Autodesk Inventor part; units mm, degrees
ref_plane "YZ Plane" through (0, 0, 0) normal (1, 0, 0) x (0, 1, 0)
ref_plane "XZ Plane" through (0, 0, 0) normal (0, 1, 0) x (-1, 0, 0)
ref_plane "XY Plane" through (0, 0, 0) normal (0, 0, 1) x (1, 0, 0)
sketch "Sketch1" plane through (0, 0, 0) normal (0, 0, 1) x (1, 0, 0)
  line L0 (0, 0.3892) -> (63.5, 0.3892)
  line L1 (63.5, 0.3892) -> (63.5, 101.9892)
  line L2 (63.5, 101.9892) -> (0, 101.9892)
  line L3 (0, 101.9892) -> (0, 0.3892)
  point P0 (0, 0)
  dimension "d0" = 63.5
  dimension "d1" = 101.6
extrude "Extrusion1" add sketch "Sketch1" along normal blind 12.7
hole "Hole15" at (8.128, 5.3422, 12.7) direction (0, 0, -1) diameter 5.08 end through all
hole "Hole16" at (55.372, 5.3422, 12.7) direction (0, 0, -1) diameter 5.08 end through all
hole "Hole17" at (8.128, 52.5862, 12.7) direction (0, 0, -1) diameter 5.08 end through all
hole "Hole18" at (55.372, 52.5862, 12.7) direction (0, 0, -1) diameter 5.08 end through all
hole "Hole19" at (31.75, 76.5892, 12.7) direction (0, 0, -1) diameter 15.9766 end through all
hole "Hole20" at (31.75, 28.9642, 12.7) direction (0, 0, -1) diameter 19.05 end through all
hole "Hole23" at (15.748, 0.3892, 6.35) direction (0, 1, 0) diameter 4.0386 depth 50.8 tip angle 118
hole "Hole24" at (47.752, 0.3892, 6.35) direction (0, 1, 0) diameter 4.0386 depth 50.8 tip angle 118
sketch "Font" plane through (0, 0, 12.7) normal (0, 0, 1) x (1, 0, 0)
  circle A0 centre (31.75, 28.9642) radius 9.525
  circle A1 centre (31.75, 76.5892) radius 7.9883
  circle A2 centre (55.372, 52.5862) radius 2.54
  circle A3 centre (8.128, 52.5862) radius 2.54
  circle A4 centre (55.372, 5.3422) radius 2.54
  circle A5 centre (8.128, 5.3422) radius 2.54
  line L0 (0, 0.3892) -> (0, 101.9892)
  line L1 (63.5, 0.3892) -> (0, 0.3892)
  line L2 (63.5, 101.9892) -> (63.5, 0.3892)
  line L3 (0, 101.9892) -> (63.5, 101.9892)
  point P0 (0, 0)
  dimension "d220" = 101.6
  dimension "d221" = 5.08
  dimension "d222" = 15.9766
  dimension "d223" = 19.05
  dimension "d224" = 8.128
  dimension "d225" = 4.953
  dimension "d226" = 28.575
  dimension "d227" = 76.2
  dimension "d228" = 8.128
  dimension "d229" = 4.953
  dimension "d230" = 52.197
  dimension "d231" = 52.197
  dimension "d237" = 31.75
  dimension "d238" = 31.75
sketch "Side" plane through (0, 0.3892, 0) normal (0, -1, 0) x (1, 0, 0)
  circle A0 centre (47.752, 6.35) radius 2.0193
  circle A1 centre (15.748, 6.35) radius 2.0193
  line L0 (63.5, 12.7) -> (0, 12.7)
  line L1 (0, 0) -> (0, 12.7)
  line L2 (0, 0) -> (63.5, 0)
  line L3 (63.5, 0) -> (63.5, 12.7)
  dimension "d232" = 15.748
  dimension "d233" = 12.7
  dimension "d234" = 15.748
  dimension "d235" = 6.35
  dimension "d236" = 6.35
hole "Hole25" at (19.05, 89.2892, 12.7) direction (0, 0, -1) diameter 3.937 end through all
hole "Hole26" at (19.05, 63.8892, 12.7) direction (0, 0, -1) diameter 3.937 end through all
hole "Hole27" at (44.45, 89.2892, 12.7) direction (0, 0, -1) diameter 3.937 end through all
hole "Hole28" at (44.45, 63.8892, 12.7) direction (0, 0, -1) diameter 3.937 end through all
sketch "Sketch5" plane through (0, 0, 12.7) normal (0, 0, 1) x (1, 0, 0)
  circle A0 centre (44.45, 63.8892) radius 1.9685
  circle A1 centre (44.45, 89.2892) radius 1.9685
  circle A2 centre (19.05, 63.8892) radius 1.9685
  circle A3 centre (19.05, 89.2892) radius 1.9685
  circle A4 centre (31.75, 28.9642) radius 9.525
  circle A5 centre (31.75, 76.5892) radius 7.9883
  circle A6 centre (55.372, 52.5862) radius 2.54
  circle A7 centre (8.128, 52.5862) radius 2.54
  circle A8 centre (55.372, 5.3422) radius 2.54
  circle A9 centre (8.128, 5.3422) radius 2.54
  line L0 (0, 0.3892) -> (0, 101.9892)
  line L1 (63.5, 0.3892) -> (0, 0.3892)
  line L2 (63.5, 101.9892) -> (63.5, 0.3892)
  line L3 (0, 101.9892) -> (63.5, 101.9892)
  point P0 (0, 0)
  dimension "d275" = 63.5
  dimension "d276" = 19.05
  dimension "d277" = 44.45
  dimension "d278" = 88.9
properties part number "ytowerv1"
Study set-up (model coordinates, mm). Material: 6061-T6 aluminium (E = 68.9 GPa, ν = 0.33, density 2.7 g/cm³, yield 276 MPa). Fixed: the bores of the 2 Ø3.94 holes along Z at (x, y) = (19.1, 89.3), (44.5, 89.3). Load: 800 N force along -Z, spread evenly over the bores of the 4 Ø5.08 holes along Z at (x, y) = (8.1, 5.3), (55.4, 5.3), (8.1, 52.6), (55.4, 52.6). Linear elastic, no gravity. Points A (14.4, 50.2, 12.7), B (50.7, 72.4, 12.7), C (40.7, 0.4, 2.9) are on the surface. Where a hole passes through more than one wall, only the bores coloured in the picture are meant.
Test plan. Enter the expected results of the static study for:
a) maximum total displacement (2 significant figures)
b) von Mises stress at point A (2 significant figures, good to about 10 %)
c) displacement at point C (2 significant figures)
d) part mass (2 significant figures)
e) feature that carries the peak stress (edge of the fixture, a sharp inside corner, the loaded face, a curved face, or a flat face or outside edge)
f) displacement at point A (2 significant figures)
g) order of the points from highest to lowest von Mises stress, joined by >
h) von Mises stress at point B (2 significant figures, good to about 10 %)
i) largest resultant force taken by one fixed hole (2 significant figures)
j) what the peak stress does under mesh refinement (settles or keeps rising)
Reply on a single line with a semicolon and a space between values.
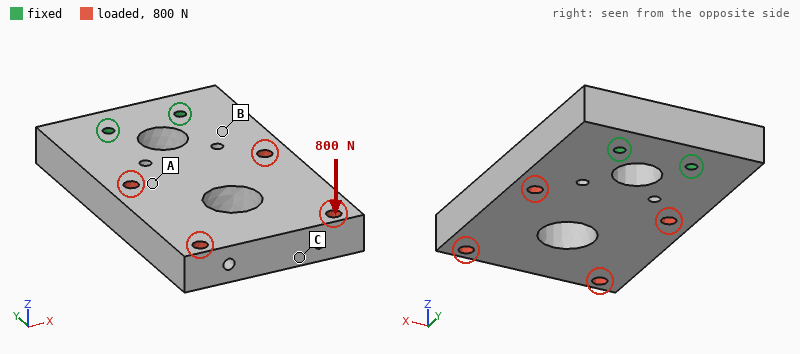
0.21 mm; 12 MPa; 0.21 mm; 200 g; edge of the fixture; 0.066 mm; B > A > C; 24 MPa; 400 N; keeps rising
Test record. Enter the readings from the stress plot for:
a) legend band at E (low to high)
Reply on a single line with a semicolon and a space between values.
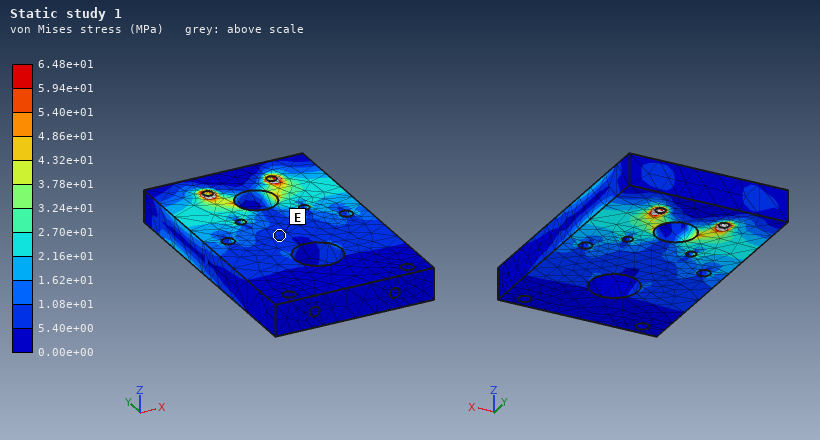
5.40e+00 to 1.08e+01 MPa
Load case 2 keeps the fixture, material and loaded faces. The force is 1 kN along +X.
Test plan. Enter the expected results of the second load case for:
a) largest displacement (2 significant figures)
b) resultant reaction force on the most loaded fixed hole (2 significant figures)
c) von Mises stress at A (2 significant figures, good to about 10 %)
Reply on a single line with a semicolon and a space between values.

31 µm; 2.1 kN; 3.2 MPa
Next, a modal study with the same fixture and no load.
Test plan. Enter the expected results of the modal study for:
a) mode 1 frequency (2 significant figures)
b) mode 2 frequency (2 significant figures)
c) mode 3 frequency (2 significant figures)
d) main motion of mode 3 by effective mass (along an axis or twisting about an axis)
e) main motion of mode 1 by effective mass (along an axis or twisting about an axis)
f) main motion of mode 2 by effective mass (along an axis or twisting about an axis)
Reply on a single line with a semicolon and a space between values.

1100 Hz; 3100 Hz; 3200 Hz; twisting about Y; along Z; along X
